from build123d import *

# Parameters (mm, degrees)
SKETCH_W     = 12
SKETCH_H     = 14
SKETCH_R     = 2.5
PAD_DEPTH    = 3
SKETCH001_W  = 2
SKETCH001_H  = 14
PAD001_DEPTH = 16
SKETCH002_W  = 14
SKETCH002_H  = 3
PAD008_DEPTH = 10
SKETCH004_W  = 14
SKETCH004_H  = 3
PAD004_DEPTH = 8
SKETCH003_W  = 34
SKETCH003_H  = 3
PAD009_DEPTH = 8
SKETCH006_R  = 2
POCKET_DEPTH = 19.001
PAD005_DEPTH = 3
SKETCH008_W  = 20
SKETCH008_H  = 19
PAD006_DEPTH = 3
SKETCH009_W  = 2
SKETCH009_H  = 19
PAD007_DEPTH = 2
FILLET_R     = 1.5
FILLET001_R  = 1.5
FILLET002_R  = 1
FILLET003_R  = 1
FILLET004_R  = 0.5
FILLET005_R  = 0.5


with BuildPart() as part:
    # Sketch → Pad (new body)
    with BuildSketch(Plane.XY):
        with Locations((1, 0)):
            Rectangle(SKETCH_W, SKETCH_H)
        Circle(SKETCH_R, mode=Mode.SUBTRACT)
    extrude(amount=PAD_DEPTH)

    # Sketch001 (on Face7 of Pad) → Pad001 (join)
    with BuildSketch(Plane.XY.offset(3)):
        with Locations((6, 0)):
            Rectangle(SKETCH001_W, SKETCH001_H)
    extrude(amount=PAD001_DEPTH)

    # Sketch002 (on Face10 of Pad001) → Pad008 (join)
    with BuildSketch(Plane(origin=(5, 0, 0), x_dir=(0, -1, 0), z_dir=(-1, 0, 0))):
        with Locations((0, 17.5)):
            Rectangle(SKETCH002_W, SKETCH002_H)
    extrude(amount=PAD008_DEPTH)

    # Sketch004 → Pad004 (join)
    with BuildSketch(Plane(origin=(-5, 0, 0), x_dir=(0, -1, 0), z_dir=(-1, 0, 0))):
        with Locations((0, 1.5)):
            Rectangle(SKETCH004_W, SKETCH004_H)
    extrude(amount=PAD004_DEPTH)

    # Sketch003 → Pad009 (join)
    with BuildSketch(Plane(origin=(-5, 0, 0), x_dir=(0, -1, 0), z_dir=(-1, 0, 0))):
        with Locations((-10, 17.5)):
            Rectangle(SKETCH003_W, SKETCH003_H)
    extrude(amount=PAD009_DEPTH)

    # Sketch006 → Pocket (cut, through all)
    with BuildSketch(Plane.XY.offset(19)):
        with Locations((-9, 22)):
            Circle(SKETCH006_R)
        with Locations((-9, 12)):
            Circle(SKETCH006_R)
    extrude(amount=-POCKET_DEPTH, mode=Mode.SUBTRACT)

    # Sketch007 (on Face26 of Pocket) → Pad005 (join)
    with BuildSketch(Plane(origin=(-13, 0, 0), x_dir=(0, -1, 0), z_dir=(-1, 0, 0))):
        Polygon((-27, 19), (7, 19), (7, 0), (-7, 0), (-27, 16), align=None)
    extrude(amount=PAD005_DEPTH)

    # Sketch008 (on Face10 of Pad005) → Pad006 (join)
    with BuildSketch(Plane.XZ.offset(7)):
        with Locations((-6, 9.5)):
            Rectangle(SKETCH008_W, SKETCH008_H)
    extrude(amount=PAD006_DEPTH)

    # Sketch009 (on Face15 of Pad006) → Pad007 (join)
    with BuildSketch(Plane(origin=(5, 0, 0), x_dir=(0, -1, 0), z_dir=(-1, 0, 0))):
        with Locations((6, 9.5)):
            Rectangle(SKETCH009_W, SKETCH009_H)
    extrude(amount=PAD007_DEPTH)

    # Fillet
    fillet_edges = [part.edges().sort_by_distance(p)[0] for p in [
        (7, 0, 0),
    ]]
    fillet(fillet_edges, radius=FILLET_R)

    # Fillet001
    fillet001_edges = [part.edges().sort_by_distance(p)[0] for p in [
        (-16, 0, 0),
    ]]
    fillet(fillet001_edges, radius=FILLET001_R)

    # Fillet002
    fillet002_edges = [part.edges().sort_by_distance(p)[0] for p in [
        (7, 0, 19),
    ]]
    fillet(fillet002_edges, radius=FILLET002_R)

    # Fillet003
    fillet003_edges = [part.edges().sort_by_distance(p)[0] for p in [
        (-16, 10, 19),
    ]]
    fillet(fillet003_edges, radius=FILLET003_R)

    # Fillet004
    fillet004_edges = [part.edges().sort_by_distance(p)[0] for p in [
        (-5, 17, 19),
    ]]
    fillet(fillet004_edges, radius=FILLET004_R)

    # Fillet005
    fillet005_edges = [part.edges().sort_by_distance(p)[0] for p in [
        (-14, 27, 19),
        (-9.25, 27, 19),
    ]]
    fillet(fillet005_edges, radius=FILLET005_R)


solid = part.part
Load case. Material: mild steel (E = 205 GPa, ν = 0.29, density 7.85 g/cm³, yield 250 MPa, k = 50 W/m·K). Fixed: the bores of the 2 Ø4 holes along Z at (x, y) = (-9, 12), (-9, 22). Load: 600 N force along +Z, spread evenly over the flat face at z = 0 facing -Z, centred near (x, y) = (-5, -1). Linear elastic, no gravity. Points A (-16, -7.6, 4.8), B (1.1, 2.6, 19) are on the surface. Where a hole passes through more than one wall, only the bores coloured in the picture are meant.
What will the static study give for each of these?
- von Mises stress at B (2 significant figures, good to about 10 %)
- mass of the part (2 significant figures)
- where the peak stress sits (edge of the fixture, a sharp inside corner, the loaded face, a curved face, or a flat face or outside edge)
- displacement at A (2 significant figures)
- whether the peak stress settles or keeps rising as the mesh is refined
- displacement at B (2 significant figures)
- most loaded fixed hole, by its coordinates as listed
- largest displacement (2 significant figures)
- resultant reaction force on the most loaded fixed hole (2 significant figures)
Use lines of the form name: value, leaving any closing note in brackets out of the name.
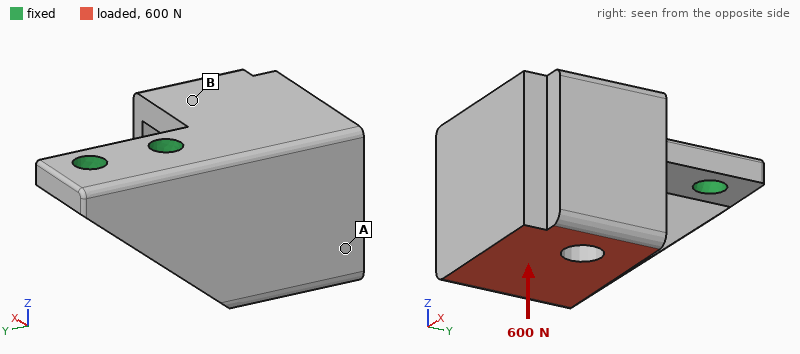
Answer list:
von Mises stress at B: 56 MPa
mass of the part: 39 g
where the peak stress sits: edge of the fixture
displacement at A: 27 µm
whether the peak stress settles or keeps rising as the mesh is refined: keeps rising
displacement at B: 38 µm
most loaded fixed hole, by its coordinates as listed: (-9, 12)
largest displacement: 70 µm
resultant reaction force on the most loaded fixed hole: 1000 N
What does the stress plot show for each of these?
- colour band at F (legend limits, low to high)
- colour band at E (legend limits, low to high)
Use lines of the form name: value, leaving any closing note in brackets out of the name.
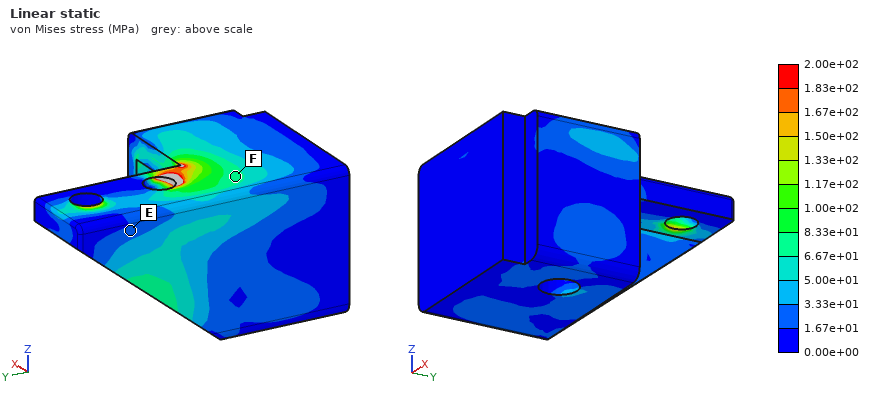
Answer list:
colour band at F: 6.67e+01 to 8.33e+01 MPa
colour band at E: 1.67e+01 to 3.33e+01 MPa
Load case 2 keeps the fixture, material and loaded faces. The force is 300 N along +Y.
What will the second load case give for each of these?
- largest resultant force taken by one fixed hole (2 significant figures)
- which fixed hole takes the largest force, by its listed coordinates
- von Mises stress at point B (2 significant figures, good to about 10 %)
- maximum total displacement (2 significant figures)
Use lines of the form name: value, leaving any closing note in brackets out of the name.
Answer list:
largest resultant force taken by one fixed hole: 430 N
which fixed hole takes the largest force, by its listed coordinates: (-9, 12)
von Mises stress at point B: 12 MPa
maximum total displacement: 36 µm
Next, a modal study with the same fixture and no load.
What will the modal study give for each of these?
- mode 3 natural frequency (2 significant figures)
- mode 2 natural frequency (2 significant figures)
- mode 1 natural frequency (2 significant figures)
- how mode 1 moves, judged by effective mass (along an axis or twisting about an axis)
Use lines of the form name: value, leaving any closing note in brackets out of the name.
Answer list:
mode 3 natural frequency: 6800 Hz
mode 2 natural frequency: 3600 Hz
mode 1 natural frequency: 2500 Hz
how mode 1 moves, judged by effective mass: along X
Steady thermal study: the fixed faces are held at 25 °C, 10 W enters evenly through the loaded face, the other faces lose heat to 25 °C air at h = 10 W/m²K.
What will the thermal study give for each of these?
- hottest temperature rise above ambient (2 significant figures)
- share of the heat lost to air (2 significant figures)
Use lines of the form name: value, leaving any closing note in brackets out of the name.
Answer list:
hottest temperature rise above ambient: 61 K
share of the heat lost to air: 13 %
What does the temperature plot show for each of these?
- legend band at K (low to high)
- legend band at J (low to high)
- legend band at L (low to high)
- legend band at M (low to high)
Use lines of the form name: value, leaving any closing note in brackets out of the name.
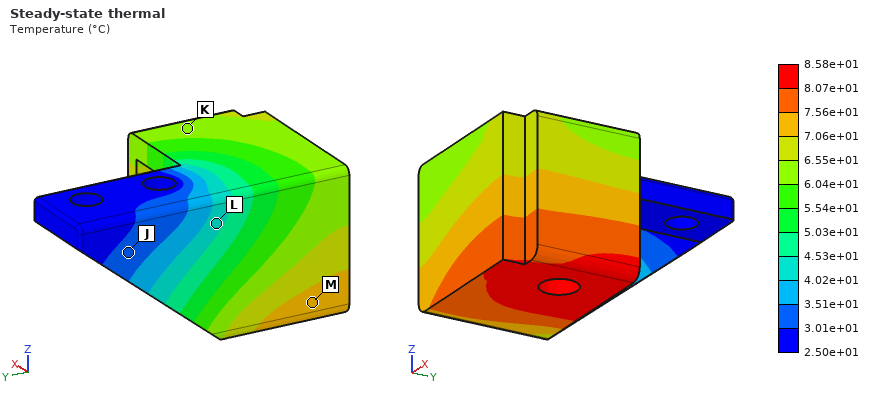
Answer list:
legend band at K: 6.04e+01 to 6.55e+01 °C
legend band at J: 3.01e+01 to 3.51e+01 °C
legend band at L: 4.02e+01 to 4.53e+01 °C
legend band at M: 7.06e+01 to 7.56e+01 °C
